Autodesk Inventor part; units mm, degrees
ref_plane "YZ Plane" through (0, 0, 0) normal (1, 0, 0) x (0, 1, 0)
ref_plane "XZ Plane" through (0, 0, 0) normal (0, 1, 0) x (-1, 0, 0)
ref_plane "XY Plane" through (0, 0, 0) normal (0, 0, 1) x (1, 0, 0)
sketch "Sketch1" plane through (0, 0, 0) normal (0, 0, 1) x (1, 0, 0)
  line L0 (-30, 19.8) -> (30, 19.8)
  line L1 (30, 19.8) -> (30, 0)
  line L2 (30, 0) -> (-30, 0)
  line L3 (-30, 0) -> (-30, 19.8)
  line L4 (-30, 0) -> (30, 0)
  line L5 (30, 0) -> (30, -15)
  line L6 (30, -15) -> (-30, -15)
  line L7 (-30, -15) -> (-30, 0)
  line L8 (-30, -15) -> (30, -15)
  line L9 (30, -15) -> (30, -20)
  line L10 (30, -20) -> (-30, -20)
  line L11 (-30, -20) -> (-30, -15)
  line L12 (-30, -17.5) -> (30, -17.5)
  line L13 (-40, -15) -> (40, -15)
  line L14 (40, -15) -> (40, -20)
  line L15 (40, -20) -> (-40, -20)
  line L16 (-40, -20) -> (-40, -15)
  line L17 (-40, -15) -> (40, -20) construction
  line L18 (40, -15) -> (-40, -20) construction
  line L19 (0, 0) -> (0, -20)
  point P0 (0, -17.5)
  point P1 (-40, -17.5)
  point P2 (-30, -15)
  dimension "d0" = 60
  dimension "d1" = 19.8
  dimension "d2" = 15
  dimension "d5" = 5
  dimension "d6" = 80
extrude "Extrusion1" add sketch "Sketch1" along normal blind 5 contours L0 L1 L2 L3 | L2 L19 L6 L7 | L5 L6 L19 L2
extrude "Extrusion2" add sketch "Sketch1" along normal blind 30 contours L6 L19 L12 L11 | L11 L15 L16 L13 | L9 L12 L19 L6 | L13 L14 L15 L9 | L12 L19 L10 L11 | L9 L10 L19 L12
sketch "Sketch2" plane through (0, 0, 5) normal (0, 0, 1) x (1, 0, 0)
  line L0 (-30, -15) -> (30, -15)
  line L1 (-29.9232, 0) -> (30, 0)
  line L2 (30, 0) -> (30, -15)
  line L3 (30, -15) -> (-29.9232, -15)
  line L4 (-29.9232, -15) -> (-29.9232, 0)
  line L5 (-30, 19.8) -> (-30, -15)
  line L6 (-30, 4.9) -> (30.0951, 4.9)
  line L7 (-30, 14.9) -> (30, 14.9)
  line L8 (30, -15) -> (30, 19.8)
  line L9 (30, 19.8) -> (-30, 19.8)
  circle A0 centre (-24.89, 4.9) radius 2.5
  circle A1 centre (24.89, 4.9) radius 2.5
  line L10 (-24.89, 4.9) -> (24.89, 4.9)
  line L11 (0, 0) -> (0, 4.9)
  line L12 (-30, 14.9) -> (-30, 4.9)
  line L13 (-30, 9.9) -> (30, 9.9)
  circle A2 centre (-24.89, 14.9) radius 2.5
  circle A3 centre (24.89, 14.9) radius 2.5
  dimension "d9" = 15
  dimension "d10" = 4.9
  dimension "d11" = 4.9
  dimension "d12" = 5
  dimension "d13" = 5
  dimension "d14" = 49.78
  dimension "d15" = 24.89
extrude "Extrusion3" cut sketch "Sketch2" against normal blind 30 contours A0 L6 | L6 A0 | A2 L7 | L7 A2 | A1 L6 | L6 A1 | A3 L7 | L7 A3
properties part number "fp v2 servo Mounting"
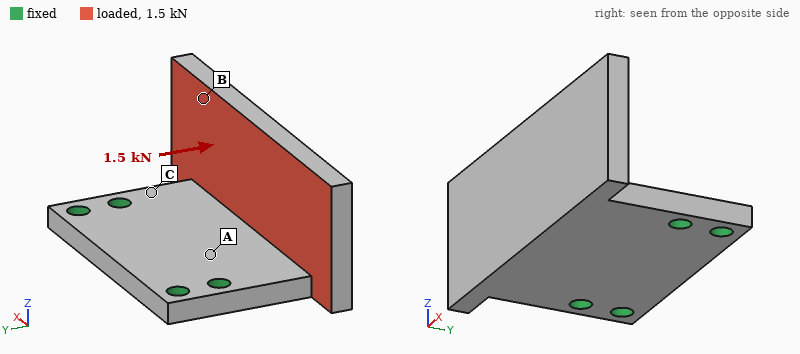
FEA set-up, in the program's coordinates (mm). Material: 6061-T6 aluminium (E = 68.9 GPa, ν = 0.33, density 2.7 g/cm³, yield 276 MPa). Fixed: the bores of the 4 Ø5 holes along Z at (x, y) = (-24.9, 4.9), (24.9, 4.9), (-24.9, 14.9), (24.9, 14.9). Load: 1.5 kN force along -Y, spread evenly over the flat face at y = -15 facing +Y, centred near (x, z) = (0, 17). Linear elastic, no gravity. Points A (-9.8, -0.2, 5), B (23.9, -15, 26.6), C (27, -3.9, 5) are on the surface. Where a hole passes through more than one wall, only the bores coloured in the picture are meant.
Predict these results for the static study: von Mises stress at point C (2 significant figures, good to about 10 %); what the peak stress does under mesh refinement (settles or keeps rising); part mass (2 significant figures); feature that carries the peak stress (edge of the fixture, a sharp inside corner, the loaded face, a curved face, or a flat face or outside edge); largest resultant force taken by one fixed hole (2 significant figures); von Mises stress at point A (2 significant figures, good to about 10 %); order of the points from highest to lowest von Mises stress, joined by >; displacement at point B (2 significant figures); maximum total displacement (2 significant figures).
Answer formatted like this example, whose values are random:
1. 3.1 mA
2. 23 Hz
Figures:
1. 110 MPa
2. keeps rising
3. 60 g
4. edge of the fixture
5. 700 N
6. 61 MPa
7. C > A > B
8. 0.34 mm
9. 0.42 mm
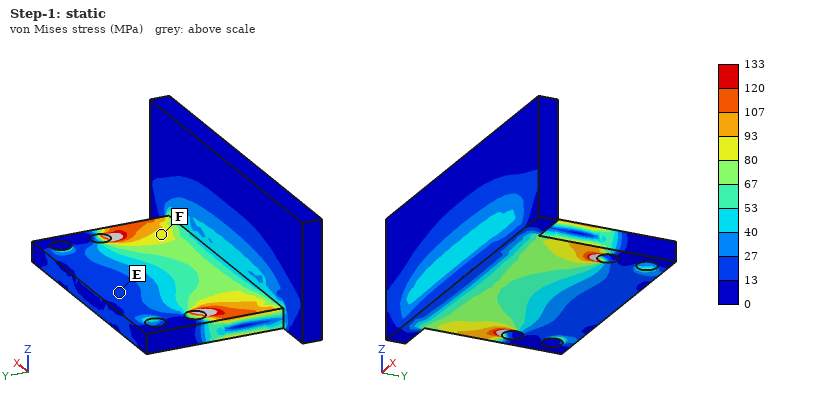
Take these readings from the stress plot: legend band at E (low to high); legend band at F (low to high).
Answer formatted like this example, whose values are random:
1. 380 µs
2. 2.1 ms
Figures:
1. 13 to 27 MPa
2. 80 to 93 MPa
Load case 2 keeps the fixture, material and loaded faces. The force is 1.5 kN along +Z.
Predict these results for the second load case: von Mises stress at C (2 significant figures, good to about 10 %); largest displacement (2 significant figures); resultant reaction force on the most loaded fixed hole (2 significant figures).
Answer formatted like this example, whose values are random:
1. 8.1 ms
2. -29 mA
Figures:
1. 95 MPa
2. 0.26 mm
3. 1.1 kN
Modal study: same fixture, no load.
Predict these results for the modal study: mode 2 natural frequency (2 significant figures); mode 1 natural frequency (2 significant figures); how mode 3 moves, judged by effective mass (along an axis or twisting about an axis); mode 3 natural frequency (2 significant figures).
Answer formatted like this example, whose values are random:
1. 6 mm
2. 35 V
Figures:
1. 2900 Hz
2. 1800 Hz
3. along Z
4. 5100 Hz
